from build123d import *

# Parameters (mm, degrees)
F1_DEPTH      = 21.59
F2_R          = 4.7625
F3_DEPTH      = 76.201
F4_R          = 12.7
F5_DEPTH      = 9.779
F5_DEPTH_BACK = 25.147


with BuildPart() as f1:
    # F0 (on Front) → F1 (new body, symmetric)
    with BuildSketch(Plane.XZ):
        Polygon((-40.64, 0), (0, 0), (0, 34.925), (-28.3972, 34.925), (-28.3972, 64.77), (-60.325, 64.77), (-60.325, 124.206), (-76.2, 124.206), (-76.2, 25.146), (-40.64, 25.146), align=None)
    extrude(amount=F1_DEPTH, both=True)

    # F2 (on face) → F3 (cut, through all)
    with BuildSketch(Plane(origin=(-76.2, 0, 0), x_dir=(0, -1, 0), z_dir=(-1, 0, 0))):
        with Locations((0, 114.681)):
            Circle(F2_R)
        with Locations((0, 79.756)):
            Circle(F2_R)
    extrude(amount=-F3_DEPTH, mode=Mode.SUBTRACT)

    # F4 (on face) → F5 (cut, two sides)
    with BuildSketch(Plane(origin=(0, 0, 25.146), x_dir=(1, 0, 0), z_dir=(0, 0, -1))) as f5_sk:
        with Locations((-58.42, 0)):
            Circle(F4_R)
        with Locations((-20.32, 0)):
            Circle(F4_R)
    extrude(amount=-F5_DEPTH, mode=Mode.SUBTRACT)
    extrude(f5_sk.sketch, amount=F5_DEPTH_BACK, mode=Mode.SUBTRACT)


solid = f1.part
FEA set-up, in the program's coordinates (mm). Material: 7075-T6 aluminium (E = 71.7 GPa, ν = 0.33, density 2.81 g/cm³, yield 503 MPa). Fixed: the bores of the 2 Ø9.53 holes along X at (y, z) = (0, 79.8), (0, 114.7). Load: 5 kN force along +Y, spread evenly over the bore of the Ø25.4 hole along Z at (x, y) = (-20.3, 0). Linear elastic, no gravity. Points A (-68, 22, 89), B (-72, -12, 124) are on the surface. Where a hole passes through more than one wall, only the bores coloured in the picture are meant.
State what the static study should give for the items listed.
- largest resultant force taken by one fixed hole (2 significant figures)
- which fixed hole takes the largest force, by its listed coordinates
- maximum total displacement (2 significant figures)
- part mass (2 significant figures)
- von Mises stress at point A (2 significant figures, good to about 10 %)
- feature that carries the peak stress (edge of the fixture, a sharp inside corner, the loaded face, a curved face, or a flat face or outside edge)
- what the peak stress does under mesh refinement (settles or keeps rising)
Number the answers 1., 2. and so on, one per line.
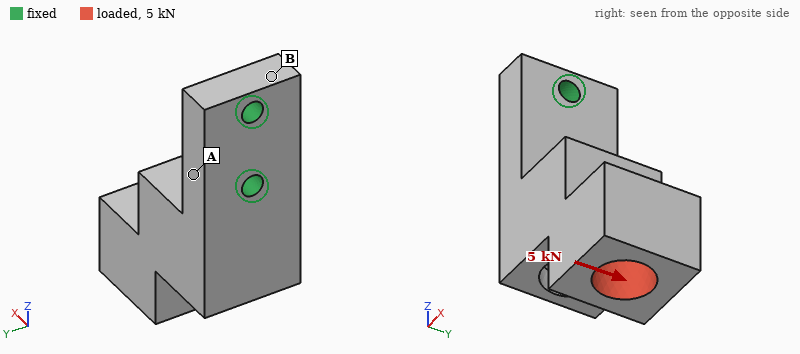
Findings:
1. 11 kN
2. (0, 79.8)
3. 0.42 mm
4. 430 g
5. 50 MPa
6. edge of the fixture
7. keeps rising
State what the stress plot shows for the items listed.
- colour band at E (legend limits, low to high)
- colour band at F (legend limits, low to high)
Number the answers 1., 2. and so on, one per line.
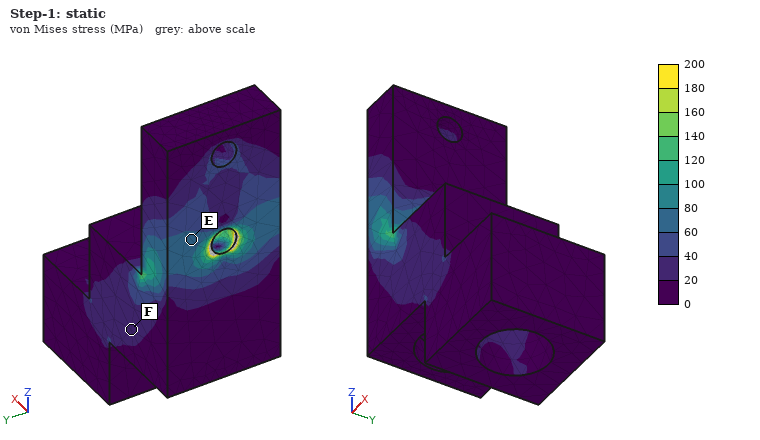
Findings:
1. 60 to 80 MPa
2. 20 to 40 MPa
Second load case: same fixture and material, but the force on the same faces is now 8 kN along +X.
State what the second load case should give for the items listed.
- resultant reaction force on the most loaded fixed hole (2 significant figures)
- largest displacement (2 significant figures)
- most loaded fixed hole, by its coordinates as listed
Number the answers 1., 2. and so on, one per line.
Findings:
1. 12 kN
2. 1.2 mm
3. (0, 79.8)
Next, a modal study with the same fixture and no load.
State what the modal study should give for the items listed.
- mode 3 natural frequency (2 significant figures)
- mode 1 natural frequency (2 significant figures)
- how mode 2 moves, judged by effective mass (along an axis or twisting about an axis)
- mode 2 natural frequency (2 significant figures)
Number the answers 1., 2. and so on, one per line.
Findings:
1. 4100 Hz
2. 1100 Hz
3. along Y
4. 1600 Hz
